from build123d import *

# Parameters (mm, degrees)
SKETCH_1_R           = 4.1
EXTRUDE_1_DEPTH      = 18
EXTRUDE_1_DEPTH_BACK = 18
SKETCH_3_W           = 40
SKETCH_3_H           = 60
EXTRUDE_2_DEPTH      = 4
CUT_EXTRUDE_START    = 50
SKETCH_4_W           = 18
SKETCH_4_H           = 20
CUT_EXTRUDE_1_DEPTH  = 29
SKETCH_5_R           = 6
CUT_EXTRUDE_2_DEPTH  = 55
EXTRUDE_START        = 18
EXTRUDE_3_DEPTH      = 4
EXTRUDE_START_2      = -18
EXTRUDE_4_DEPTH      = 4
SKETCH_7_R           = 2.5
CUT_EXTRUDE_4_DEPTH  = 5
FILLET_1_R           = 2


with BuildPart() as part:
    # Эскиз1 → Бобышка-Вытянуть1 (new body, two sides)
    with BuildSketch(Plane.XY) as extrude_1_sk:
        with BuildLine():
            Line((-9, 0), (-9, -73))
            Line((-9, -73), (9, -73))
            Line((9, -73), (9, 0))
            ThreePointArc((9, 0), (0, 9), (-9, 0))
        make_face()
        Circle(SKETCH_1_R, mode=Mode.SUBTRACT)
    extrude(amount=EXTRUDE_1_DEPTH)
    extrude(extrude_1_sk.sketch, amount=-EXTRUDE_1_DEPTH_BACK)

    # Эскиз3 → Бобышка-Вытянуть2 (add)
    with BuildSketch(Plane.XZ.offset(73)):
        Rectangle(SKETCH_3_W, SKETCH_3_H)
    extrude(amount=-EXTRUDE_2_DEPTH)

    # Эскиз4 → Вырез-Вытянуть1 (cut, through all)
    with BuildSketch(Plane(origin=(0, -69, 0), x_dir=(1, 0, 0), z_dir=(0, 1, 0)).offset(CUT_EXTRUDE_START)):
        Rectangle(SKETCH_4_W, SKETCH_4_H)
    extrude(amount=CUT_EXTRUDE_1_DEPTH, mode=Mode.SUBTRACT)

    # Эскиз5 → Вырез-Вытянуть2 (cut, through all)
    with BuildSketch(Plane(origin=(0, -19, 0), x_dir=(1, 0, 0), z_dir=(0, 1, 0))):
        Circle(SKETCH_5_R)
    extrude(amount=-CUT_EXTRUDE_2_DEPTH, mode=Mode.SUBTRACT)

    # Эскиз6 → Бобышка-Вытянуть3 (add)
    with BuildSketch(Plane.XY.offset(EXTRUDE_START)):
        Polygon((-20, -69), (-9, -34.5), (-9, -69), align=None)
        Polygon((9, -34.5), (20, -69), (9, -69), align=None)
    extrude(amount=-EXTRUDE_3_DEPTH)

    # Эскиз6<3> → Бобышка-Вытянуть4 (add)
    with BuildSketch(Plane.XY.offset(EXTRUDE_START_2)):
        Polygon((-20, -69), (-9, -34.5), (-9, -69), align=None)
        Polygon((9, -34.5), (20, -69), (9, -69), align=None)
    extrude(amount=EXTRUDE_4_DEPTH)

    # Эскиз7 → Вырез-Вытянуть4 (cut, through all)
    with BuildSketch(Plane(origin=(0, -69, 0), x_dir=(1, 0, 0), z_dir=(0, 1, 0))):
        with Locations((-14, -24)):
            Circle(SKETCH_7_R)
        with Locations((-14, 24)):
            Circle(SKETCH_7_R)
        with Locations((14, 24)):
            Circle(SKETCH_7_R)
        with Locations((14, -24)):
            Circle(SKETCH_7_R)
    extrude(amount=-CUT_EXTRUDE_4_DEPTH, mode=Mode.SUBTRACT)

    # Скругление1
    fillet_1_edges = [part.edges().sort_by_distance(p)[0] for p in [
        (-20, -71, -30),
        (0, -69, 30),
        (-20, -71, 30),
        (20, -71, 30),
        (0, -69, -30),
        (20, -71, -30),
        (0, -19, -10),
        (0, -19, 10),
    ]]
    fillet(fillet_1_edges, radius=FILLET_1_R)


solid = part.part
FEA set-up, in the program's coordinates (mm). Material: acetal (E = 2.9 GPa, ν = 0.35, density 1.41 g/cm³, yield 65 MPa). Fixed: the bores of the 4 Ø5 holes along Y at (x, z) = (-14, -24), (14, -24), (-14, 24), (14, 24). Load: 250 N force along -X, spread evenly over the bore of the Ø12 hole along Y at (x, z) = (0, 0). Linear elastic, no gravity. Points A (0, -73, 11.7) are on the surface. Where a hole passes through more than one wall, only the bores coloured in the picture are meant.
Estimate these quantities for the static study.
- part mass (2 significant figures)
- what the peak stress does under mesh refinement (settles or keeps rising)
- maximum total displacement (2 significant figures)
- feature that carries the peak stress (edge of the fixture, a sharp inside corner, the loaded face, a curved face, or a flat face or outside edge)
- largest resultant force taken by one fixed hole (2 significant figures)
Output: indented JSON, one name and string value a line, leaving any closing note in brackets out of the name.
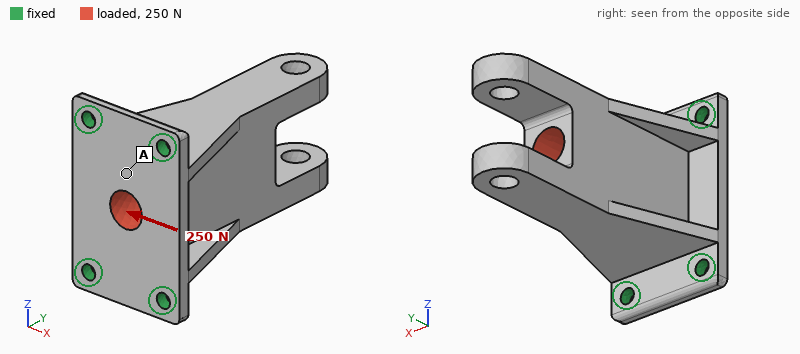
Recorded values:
{
  "part mass": "64 g",
  "what the peak stress does under mesh refinement": "keeps rising",
  "maximum total displacement": "0.27 mm",
  "feature that carries the peak stress": "edge of the fixture",
  "largest resultant force taken by one fixed hole": "130 N"
}
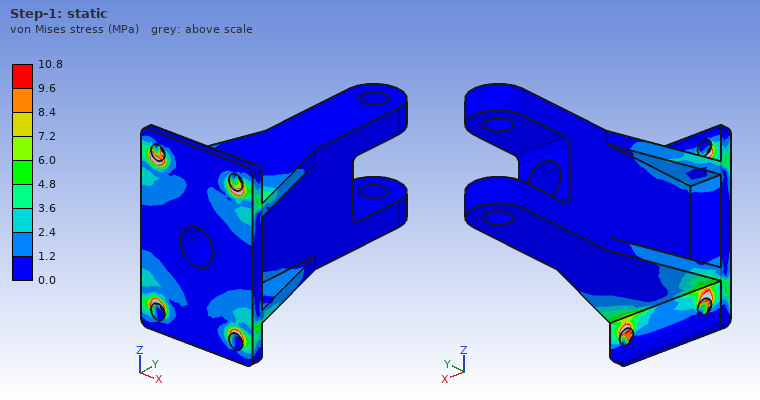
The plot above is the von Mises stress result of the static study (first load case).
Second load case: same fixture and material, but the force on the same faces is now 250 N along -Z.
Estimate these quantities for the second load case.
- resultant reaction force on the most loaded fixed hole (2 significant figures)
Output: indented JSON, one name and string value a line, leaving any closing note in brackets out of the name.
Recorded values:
{
  "resultant reaction force on the most loaded fixed hole": "100 N"
}
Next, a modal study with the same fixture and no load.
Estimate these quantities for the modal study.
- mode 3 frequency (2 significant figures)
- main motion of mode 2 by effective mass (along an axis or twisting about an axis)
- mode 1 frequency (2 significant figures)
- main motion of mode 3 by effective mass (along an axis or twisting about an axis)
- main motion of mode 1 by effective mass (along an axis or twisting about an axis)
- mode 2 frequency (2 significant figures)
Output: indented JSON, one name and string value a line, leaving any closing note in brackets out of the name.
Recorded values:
{
  "mode 3 frequency": "1900 Hz",
  "main motion of mode 2 by effective mass": "along Z",
  "mode 1 frequency": "750 Hz",
  "main motion of mode 3 by effective mass": "twisting about Y",
  "main motion of mode 1 by effective mass": "along X",
  "mode 2 frequency": "1000 Hz"
}
